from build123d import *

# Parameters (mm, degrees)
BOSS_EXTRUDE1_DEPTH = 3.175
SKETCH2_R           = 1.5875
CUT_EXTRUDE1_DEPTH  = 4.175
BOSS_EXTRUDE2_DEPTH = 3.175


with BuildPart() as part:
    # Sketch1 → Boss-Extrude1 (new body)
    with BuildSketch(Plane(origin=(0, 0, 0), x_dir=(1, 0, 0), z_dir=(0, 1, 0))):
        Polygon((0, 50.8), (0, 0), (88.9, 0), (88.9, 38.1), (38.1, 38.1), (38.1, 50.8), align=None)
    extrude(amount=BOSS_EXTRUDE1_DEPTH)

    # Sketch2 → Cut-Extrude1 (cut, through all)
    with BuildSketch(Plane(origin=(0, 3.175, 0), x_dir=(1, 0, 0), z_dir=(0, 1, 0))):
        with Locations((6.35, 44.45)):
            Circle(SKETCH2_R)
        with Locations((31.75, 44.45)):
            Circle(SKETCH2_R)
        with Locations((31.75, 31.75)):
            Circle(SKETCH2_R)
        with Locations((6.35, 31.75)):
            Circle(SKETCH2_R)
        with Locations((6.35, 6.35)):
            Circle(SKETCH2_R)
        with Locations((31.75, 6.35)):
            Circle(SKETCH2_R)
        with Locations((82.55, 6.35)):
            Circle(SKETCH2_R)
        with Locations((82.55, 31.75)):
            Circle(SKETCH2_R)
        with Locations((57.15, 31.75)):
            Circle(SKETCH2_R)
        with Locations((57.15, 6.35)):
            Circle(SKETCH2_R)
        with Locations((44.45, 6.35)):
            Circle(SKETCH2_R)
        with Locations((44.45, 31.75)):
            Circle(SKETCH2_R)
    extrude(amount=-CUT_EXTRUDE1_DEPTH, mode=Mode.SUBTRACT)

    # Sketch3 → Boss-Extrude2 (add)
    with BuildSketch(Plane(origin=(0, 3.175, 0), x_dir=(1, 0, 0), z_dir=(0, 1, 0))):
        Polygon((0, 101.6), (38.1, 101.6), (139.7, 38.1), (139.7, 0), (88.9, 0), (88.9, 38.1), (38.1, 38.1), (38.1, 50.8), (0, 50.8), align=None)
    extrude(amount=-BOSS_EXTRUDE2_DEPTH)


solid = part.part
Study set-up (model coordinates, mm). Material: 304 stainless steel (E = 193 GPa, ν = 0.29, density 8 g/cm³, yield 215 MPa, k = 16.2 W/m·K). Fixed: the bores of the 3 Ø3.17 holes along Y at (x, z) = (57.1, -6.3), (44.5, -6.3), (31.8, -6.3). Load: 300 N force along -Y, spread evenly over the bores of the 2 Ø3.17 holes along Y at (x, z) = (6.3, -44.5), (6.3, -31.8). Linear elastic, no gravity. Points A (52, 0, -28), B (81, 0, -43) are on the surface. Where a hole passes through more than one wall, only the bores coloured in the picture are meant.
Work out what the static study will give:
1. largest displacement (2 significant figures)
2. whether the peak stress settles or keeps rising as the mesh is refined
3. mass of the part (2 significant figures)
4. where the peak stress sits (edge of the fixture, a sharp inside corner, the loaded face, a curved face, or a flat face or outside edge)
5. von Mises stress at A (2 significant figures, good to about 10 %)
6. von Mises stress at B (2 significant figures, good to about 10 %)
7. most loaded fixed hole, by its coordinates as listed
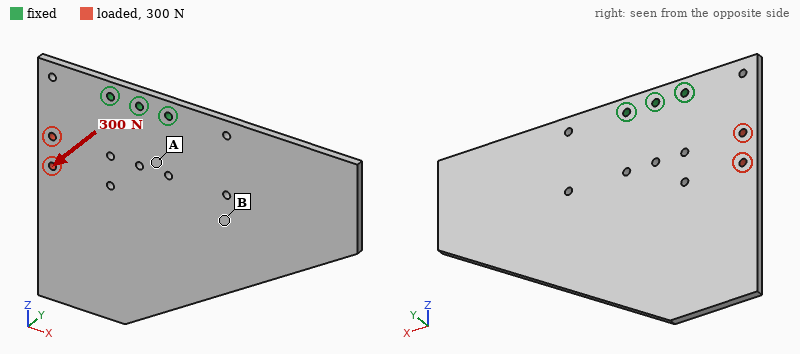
0.62 mm
keeps rising
280 g
edge of the fixture
52 MPa
18 MPa
(31.8, -6.3)
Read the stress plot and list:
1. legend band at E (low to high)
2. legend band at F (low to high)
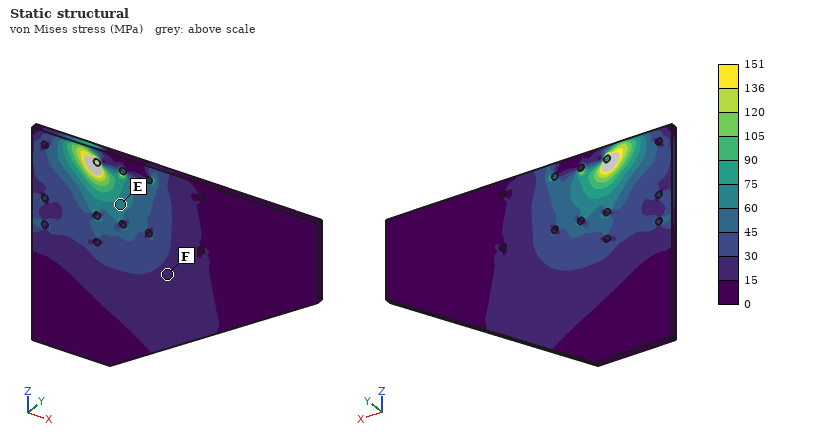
60 to 75 MPa
15 to 30 MPa
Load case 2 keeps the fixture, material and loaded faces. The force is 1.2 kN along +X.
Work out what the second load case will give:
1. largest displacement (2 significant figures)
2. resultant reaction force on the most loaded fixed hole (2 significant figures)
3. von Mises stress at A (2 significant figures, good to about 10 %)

26 µm
1.4 kN
13 MPa
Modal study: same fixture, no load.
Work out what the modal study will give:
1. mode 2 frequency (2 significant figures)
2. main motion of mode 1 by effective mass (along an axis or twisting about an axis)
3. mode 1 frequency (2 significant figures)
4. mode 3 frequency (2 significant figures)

340 Hz
along Y
290 Hz
790 Hz
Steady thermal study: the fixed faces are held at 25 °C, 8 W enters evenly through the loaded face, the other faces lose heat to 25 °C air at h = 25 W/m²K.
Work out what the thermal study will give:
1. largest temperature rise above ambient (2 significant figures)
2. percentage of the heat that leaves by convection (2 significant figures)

82 K
77 %
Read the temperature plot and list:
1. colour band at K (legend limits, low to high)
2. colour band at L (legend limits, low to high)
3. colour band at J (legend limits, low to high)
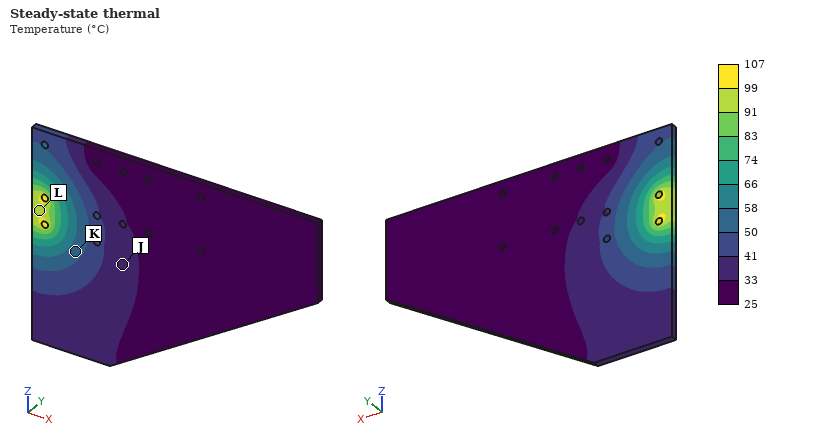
50 to 58 °C
91 to 99 °C
33 to 41 °C
